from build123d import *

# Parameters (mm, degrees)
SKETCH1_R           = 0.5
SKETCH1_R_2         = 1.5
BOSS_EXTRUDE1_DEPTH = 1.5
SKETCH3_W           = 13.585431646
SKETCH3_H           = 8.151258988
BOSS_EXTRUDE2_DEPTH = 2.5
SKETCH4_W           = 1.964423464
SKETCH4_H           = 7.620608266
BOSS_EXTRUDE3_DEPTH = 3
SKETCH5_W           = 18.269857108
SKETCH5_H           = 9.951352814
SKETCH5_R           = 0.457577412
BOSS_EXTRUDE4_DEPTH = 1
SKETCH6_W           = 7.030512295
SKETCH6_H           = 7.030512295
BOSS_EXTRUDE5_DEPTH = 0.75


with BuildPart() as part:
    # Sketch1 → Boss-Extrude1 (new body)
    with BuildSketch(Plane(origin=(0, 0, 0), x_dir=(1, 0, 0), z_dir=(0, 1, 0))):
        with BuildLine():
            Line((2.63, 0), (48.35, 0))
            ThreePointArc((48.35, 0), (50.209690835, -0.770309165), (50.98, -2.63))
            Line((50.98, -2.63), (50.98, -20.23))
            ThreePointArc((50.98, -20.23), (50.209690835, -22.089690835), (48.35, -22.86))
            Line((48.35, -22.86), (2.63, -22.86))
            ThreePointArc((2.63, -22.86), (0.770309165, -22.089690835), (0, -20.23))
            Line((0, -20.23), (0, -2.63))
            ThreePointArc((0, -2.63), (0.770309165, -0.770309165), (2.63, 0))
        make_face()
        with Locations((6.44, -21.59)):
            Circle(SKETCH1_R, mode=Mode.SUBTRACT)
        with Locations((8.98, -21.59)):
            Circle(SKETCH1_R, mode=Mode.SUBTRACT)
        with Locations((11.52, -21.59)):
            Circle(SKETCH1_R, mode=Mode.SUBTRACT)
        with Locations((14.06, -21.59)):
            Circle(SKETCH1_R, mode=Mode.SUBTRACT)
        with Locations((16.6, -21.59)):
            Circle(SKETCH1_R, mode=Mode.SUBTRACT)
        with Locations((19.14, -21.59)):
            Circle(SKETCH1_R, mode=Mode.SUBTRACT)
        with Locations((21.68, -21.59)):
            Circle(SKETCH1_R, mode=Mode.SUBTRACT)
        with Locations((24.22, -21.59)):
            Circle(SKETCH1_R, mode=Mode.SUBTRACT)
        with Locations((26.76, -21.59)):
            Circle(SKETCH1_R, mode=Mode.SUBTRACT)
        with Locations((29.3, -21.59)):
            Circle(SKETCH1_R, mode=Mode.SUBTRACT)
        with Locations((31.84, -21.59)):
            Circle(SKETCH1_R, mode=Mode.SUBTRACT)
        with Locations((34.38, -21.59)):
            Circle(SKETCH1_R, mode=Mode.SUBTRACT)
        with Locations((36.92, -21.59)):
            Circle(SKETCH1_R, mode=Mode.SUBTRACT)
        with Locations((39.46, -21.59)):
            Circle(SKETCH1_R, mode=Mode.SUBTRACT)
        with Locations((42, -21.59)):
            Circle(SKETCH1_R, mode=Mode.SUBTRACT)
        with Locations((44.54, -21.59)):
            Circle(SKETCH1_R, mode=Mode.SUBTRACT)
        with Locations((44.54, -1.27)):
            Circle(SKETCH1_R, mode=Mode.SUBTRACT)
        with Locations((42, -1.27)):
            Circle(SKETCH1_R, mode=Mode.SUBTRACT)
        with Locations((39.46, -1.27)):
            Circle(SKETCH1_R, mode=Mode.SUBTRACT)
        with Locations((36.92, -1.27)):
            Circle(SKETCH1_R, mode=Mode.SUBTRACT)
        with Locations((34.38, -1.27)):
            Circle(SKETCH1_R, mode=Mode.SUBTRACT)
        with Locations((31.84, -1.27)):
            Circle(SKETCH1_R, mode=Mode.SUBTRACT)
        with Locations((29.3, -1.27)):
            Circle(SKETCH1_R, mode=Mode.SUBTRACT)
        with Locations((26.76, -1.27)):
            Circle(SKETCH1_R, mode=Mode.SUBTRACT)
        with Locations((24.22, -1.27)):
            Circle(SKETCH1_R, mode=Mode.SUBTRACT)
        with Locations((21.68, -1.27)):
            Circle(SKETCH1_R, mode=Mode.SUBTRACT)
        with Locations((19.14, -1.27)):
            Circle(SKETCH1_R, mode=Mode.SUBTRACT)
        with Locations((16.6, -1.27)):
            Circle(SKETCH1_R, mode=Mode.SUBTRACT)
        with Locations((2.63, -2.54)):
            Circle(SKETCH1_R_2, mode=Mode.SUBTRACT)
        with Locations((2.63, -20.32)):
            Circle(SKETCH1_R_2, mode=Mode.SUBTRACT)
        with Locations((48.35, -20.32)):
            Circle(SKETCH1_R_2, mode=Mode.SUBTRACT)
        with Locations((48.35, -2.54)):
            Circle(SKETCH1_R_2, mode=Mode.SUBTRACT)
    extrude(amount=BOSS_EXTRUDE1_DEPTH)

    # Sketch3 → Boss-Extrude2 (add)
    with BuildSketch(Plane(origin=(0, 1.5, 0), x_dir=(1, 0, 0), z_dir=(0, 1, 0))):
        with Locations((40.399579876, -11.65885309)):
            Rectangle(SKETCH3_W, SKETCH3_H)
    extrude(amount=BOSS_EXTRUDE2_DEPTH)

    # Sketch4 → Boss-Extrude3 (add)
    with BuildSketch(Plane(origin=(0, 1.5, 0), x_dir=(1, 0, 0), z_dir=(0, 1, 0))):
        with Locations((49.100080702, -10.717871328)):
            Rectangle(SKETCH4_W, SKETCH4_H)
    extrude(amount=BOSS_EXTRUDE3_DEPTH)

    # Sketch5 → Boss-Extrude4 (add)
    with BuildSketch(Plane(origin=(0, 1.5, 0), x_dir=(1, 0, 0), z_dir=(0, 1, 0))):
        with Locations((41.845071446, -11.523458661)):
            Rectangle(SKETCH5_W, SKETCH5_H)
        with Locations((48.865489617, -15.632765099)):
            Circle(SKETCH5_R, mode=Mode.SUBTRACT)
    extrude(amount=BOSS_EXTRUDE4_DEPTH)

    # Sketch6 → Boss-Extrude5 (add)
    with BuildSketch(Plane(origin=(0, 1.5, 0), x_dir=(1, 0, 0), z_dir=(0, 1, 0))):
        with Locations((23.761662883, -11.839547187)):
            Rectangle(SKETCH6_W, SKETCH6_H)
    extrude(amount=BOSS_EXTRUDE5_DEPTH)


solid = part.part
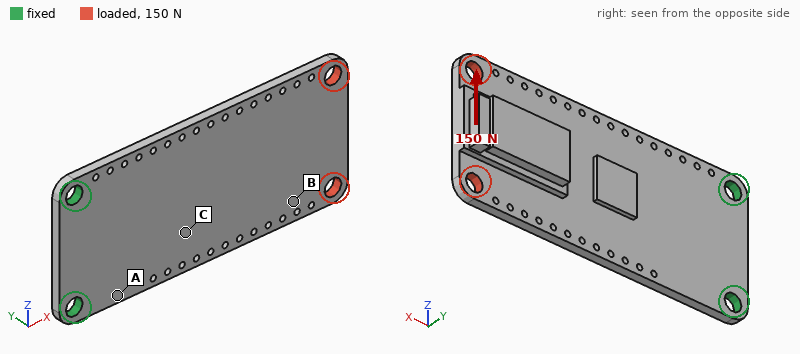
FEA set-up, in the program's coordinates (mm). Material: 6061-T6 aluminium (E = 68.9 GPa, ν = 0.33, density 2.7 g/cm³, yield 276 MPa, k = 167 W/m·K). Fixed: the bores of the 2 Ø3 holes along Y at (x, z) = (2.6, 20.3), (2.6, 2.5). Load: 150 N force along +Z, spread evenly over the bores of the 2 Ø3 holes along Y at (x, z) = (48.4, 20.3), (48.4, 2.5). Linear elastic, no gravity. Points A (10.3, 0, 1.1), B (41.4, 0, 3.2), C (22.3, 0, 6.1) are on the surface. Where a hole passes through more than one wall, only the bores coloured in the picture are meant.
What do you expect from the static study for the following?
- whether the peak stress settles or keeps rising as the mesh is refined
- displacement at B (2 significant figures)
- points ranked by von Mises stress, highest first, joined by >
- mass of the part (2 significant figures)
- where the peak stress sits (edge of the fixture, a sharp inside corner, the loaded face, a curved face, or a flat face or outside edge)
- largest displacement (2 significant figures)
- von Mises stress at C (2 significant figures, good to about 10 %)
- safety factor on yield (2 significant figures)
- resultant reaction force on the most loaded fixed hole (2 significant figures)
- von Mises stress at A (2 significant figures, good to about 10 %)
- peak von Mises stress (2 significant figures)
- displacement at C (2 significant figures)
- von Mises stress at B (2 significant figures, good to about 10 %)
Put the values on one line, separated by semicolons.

settles; 48 µm; A > C > B; 5.6 g; a curved face; 67 µm; 18 MPa; 2.6; 380 N; 40 MPa; 110 MPa; 16 µm; 8.8 MPa
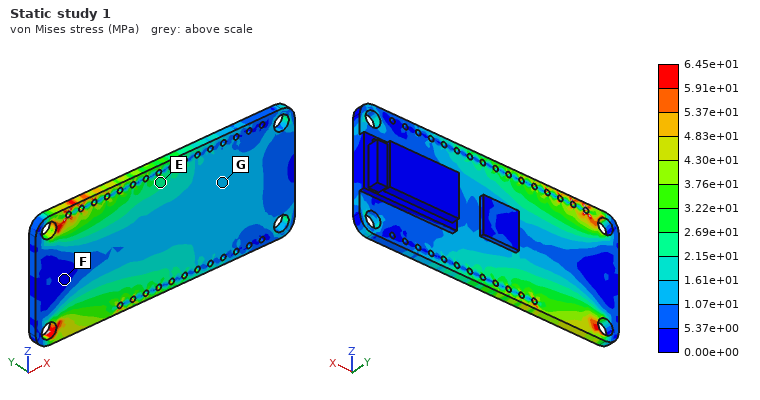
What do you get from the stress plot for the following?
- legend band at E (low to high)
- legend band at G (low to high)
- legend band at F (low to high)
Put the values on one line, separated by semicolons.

2.15e+01 to 2.69e+01 MPa; 1.07e+01 to 1.61e+01 MPa; 0.00e+00 to 5.37e+00 MPa
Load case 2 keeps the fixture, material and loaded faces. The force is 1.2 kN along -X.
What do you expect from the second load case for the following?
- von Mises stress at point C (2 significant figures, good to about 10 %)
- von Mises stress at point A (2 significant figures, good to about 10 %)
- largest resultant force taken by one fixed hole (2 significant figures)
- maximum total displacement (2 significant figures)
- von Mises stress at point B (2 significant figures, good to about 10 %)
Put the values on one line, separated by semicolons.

43 MPa; 42 MPa; 620 N; 65 µm; 54 MPa
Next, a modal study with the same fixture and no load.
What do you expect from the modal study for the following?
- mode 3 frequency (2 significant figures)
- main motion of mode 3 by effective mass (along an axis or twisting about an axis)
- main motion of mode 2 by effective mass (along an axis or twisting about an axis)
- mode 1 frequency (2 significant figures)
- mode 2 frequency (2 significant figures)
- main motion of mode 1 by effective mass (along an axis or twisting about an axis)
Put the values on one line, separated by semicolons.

3400 Hz; along Y; twisting about X; 440 Hz; 2700 Hz; along Y
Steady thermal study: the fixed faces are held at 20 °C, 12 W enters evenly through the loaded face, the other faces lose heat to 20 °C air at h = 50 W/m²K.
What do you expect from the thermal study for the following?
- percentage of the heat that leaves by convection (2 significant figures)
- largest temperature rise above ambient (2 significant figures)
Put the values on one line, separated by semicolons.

39 %; 77 K
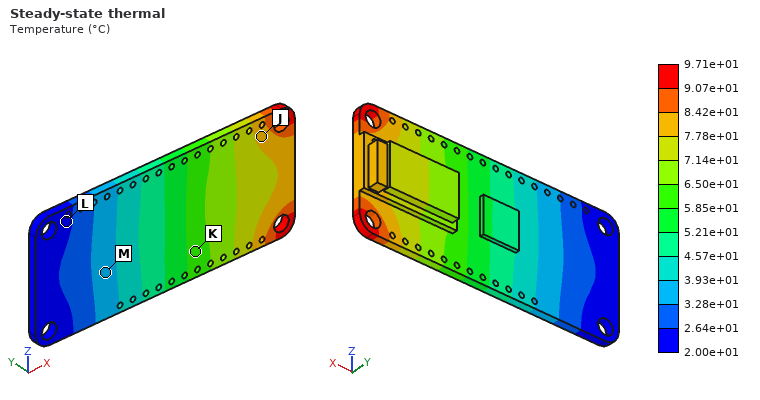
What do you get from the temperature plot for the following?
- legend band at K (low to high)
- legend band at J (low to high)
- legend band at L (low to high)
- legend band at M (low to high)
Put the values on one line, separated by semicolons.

5.85e+01 to 6.50e+01 °C; 7.78e+01 to 8.42e+01 °C; 2.00e+01 to 2.64e+01 °C; 3.28e+01 to 3.93e+01 °C
